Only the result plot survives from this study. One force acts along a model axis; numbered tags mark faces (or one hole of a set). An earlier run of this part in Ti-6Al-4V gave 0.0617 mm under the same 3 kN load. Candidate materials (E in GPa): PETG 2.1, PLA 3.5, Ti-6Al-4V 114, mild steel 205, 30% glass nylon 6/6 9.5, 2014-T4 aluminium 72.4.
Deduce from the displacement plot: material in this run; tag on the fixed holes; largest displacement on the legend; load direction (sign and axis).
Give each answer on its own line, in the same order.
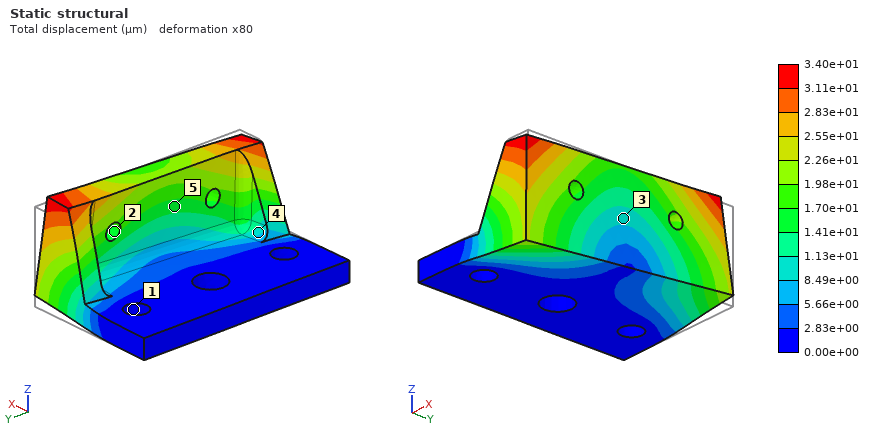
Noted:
mild steel
1
3.40e+01 µm
-Y
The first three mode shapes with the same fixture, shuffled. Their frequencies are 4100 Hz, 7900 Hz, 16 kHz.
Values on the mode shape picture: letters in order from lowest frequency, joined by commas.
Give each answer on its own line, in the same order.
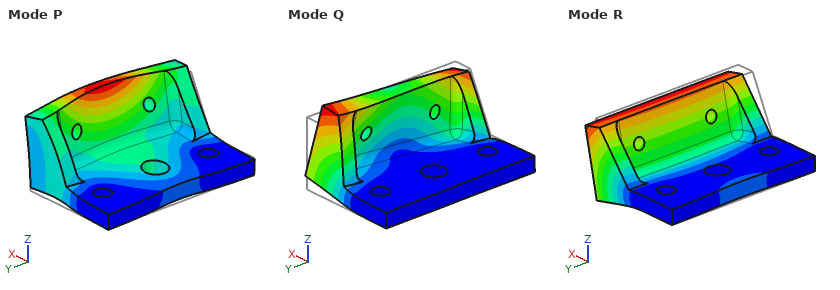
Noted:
R, Q, P
